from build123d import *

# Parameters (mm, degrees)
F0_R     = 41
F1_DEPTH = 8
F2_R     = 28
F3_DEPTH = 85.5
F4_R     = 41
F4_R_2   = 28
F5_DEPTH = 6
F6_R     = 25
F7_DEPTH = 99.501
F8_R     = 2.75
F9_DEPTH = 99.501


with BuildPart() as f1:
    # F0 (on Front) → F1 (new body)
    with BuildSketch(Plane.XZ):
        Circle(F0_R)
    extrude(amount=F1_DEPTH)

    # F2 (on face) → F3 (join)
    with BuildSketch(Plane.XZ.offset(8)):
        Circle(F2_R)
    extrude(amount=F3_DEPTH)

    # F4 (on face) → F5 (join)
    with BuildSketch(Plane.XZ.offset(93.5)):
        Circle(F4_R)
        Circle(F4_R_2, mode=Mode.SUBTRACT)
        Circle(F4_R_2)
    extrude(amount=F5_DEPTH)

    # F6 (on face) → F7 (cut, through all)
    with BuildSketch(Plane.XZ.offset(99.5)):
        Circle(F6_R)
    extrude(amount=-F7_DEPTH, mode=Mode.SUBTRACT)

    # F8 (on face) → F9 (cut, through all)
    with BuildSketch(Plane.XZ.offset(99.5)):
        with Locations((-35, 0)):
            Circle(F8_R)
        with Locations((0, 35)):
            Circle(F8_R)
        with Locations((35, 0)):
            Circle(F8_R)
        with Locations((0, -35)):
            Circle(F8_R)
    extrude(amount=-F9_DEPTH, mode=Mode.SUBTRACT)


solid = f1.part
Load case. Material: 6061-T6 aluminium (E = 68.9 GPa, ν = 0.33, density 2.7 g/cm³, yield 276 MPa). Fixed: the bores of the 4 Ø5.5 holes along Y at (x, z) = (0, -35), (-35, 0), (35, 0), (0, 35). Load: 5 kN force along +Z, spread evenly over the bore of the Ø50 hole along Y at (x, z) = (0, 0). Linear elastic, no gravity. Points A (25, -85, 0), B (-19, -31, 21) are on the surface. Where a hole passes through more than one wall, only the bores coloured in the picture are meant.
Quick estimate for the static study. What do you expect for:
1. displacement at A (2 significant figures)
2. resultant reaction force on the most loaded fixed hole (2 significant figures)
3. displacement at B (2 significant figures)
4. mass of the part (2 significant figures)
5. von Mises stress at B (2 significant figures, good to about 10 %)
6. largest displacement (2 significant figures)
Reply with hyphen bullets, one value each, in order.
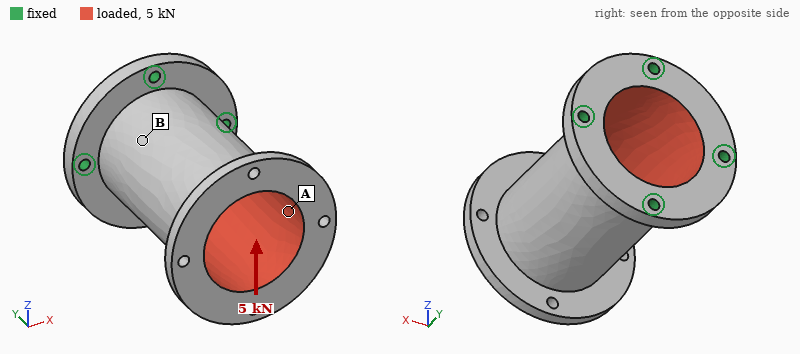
- 0.11 mm
- 3.7 kN
- 0.045 mm
- 240 g
- 22 MPa
- 0.14 mm
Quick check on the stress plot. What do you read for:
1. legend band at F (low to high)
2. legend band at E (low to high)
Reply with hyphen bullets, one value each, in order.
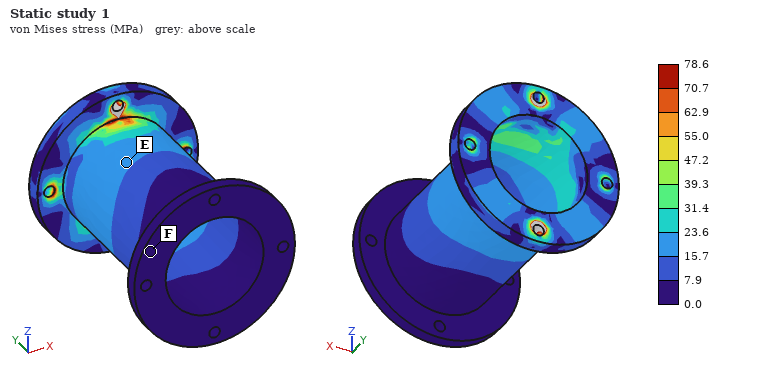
- 0.0 to 7.9 MPa
- 15.7 to 23.6 MPa
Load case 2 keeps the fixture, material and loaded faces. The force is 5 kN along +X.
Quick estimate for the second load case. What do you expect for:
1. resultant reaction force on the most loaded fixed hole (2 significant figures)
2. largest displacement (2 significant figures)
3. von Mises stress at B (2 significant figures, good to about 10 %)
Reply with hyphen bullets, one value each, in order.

- 3.7 kN
- 0.14 mm
- 22 MPa
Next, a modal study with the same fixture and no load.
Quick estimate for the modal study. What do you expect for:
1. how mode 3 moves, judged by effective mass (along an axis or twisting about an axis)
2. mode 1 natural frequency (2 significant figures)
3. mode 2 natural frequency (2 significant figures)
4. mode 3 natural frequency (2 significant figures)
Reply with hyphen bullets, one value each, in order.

- twisting about Y
- 2200 Hz
- 2200 Hz
- 5300 Hz
